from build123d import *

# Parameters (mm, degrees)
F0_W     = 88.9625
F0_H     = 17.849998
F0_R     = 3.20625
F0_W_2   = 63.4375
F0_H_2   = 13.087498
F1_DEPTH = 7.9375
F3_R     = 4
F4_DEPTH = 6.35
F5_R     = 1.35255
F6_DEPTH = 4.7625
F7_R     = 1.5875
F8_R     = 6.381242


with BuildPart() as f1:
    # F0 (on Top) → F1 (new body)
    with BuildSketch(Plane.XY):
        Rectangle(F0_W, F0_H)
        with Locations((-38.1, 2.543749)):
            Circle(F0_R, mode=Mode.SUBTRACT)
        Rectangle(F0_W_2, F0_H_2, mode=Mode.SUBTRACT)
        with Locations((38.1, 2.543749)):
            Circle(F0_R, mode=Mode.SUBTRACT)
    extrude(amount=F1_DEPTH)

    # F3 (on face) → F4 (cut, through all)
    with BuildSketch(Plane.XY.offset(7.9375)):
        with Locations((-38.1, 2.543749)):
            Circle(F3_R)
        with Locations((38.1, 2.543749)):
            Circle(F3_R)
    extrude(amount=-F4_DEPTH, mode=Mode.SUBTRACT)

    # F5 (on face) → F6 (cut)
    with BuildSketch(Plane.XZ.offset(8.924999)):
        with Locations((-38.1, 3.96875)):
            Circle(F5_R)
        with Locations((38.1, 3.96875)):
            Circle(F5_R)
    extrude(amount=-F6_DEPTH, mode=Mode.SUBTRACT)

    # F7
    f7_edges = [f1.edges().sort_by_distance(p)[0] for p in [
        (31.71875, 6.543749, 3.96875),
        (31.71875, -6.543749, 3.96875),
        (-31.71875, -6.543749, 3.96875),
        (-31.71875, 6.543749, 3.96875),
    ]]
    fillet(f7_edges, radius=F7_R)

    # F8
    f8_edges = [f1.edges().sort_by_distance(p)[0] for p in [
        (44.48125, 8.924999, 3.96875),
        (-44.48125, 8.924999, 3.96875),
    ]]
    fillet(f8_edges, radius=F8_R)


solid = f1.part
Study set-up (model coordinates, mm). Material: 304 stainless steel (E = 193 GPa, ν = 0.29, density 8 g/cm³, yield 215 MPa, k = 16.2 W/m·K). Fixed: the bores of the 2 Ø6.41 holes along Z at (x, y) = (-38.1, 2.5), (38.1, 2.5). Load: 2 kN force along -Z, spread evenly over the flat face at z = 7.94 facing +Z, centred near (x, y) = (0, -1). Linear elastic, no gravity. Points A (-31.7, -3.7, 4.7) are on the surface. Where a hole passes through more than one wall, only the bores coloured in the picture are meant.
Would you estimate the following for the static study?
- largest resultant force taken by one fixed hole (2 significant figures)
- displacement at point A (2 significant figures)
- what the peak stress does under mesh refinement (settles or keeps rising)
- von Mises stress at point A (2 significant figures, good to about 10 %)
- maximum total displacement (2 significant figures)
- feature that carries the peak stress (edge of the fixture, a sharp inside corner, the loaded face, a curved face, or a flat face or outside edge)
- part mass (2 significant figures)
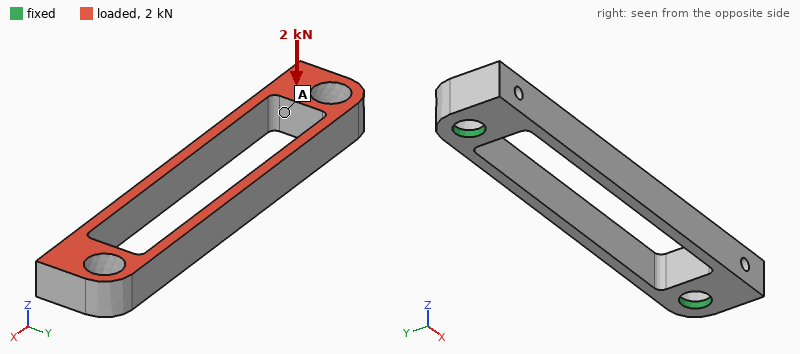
1.1 kN
9.7 µm
keeps rising
45 MPa
52 µm
edge of the fixture
41 g
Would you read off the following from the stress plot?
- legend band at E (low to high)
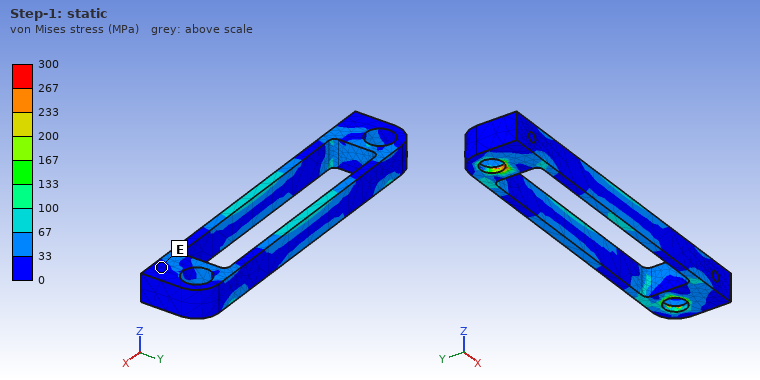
0 to 33 MPa
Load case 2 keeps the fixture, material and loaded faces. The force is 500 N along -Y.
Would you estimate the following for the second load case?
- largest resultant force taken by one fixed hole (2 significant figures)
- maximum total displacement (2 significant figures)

250 N
60 µm
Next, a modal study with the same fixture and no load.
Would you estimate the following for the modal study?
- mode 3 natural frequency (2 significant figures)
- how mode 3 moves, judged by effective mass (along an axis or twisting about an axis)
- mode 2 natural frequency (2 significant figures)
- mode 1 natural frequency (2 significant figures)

5800 Hz
along Z
2800 Hz
2800 Hz
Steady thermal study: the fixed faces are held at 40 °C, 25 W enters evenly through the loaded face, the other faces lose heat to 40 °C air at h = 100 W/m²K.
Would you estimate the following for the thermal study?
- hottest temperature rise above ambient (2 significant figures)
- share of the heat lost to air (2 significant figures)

55 K
55 %
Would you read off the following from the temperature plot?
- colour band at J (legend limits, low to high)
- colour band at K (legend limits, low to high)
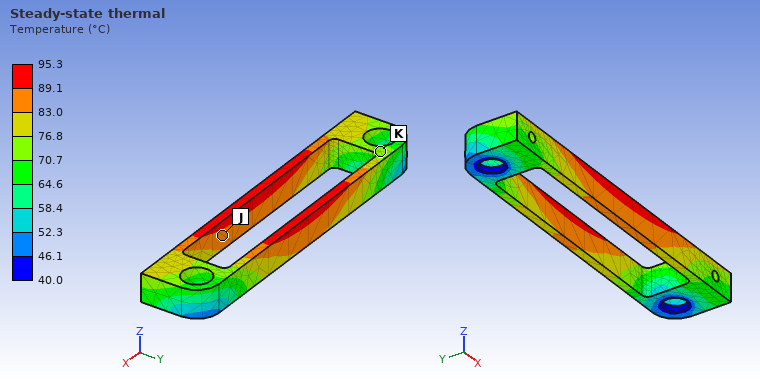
83.0 to 89.1 °C
70.7 to 76.8 °C
